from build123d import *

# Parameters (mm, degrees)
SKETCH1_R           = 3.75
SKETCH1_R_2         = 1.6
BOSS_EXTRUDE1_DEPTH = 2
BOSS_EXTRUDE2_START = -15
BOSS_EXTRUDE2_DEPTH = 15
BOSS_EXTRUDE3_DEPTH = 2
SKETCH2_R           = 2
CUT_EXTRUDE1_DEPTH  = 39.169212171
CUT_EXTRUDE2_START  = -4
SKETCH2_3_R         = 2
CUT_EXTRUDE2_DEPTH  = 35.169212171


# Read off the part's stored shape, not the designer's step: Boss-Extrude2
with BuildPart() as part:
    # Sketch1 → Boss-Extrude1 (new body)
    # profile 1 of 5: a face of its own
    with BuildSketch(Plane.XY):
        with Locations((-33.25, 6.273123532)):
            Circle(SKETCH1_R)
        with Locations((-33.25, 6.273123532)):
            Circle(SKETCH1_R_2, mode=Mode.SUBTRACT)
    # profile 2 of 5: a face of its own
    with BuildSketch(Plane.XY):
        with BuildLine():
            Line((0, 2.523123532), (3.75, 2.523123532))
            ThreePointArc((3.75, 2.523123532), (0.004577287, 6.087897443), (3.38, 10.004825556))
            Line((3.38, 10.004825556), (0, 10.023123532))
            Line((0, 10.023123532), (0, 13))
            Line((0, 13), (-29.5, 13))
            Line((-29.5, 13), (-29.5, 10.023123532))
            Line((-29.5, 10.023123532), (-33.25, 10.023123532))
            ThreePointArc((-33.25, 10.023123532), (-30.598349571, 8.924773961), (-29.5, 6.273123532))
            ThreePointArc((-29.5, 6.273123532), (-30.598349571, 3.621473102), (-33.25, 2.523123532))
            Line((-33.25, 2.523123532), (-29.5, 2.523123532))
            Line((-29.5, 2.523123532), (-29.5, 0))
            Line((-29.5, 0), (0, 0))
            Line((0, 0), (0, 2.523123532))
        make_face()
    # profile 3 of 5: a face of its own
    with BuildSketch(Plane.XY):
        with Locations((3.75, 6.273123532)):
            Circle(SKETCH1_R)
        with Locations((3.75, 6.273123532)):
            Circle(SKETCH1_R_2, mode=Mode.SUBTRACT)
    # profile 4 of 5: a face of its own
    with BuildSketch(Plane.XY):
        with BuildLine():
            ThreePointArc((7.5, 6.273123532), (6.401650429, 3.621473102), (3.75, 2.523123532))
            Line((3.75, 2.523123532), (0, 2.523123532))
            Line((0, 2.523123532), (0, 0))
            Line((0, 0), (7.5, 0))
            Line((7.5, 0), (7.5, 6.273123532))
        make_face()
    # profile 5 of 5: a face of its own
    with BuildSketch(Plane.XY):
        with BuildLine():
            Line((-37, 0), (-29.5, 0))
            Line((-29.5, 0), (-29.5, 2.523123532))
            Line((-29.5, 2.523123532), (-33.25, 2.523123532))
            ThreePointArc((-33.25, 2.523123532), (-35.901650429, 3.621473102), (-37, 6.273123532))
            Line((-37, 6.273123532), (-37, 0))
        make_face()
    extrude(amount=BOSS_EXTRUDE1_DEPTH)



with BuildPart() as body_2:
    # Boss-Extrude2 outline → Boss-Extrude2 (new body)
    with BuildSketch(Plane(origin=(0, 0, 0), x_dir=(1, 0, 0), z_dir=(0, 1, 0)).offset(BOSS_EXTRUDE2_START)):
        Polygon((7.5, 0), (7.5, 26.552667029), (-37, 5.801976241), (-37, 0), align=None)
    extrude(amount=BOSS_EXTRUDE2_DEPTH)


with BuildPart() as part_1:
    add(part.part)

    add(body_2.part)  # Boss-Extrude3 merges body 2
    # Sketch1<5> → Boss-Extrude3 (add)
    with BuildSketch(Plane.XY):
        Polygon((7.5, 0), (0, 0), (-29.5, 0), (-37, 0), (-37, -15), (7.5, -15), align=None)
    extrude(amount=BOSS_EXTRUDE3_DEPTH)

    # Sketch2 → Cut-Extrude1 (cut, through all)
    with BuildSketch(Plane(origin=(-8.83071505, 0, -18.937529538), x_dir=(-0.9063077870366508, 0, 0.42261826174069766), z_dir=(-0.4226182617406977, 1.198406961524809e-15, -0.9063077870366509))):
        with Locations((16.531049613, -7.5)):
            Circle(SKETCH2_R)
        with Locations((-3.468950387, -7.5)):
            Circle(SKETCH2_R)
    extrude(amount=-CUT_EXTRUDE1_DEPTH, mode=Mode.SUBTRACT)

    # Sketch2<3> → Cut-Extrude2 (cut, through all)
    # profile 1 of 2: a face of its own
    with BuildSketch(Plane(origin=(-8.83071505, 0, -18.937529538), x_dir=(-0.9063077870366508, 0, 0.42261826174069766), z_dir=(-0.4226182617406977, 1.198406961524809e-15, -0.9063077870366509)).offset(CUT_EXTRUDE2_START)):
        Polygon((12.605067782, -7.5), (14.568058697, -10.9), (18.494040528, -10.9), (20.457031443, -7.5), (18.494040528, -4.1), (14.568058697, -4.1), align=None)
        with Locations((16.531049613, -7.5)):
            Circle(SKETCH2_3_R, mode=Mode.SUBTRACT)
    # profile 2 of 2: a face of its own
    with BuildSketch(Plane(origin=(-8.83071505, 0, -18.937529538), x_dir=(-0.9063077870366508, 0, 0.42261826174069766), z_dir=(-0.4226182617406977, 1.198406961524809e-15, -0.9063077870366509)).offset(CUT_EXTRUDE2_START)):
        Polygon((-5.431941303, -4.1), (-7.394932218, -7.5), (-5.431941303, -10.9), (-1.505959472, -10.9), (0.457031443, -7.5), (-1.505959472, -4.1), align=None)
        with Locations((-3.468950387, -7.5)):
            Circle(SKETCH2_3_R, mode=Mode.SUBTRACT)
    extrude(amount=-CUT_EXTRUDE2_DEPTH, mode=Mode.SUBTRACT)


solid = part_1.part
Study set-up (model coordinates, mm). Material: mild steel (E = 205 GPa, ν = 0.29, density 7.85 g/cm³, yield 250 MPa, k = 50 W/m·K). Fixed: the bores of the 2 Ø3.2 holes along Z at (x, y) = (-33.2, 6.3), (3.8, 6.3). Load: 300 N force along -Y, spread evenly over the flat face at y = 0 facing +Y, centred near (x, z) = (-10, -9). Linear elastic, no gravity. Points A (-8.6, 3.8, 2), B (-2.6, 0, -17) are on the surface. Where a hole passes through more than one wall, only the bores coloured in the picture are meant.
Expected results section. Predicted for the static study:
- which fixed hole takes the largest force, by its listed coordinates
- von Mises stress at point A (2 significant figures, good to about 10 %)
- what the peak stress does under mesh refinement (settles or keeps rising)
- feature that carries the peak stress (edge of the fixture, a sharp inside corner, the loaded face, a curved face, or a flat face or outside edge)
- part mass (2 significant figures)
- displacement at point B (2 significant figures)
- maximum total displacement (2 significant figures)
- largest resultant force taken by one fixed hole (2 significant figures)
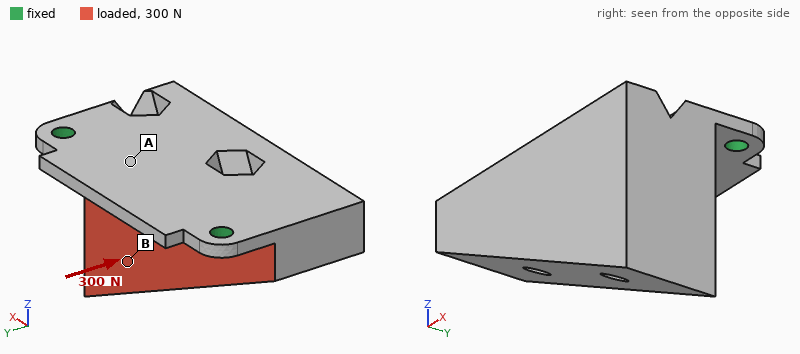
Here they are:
(3.8, 6.3)
54 MPa
keeps rising
edge of the fixture
92 g
0.086 mm
0.15 mm
190 N
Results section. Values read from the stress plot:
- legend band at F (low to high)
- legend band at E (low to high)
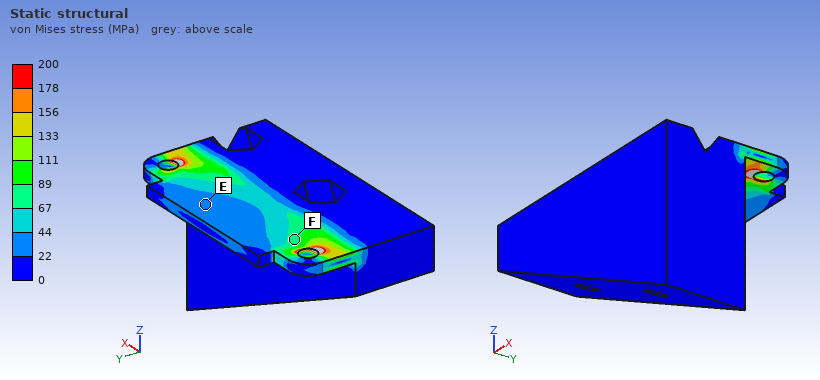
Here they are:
67 to 89 MPa
22 to 44 MPa
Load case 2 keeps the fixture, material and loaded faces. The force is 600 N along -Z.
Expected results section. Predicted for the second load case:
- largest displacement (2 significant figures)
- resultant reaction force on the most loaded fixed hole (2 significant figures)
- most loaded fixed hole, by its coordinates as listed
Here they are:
85 µm
380 N
(3.8, 6.3)
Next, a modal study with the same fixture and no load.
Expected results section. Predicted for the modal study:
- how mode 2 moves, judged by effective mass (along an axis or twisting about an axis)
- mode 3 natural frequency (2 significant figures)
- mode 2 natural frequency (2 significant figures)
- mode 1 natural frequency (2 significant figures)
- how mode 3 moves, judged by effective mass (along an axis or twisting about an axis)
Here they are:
along X
6400 Hz
5000 Hz
870 Hz
along Z
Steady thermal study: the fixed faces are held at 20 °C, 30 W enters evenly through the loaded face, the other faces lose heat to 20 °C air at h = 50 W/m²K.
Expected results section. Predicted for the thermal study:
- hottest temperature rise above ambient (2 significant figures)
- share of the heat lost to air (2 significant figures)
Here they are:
72 K
41 %
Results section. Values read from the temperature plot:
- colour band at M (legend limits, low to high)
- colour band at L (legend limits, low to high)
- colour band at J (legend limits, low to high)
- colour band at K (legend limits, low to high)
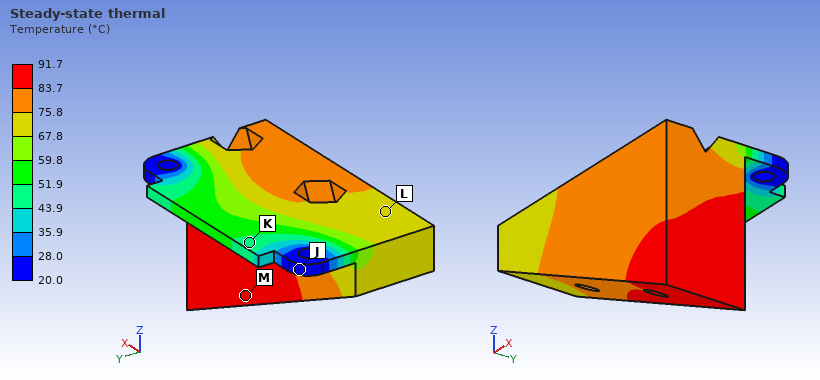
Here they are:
83.7 to 91.7 °C
67.8 to 75.8 °C
20.0 to 28.0 °C
43.9 to 51.9 °C
